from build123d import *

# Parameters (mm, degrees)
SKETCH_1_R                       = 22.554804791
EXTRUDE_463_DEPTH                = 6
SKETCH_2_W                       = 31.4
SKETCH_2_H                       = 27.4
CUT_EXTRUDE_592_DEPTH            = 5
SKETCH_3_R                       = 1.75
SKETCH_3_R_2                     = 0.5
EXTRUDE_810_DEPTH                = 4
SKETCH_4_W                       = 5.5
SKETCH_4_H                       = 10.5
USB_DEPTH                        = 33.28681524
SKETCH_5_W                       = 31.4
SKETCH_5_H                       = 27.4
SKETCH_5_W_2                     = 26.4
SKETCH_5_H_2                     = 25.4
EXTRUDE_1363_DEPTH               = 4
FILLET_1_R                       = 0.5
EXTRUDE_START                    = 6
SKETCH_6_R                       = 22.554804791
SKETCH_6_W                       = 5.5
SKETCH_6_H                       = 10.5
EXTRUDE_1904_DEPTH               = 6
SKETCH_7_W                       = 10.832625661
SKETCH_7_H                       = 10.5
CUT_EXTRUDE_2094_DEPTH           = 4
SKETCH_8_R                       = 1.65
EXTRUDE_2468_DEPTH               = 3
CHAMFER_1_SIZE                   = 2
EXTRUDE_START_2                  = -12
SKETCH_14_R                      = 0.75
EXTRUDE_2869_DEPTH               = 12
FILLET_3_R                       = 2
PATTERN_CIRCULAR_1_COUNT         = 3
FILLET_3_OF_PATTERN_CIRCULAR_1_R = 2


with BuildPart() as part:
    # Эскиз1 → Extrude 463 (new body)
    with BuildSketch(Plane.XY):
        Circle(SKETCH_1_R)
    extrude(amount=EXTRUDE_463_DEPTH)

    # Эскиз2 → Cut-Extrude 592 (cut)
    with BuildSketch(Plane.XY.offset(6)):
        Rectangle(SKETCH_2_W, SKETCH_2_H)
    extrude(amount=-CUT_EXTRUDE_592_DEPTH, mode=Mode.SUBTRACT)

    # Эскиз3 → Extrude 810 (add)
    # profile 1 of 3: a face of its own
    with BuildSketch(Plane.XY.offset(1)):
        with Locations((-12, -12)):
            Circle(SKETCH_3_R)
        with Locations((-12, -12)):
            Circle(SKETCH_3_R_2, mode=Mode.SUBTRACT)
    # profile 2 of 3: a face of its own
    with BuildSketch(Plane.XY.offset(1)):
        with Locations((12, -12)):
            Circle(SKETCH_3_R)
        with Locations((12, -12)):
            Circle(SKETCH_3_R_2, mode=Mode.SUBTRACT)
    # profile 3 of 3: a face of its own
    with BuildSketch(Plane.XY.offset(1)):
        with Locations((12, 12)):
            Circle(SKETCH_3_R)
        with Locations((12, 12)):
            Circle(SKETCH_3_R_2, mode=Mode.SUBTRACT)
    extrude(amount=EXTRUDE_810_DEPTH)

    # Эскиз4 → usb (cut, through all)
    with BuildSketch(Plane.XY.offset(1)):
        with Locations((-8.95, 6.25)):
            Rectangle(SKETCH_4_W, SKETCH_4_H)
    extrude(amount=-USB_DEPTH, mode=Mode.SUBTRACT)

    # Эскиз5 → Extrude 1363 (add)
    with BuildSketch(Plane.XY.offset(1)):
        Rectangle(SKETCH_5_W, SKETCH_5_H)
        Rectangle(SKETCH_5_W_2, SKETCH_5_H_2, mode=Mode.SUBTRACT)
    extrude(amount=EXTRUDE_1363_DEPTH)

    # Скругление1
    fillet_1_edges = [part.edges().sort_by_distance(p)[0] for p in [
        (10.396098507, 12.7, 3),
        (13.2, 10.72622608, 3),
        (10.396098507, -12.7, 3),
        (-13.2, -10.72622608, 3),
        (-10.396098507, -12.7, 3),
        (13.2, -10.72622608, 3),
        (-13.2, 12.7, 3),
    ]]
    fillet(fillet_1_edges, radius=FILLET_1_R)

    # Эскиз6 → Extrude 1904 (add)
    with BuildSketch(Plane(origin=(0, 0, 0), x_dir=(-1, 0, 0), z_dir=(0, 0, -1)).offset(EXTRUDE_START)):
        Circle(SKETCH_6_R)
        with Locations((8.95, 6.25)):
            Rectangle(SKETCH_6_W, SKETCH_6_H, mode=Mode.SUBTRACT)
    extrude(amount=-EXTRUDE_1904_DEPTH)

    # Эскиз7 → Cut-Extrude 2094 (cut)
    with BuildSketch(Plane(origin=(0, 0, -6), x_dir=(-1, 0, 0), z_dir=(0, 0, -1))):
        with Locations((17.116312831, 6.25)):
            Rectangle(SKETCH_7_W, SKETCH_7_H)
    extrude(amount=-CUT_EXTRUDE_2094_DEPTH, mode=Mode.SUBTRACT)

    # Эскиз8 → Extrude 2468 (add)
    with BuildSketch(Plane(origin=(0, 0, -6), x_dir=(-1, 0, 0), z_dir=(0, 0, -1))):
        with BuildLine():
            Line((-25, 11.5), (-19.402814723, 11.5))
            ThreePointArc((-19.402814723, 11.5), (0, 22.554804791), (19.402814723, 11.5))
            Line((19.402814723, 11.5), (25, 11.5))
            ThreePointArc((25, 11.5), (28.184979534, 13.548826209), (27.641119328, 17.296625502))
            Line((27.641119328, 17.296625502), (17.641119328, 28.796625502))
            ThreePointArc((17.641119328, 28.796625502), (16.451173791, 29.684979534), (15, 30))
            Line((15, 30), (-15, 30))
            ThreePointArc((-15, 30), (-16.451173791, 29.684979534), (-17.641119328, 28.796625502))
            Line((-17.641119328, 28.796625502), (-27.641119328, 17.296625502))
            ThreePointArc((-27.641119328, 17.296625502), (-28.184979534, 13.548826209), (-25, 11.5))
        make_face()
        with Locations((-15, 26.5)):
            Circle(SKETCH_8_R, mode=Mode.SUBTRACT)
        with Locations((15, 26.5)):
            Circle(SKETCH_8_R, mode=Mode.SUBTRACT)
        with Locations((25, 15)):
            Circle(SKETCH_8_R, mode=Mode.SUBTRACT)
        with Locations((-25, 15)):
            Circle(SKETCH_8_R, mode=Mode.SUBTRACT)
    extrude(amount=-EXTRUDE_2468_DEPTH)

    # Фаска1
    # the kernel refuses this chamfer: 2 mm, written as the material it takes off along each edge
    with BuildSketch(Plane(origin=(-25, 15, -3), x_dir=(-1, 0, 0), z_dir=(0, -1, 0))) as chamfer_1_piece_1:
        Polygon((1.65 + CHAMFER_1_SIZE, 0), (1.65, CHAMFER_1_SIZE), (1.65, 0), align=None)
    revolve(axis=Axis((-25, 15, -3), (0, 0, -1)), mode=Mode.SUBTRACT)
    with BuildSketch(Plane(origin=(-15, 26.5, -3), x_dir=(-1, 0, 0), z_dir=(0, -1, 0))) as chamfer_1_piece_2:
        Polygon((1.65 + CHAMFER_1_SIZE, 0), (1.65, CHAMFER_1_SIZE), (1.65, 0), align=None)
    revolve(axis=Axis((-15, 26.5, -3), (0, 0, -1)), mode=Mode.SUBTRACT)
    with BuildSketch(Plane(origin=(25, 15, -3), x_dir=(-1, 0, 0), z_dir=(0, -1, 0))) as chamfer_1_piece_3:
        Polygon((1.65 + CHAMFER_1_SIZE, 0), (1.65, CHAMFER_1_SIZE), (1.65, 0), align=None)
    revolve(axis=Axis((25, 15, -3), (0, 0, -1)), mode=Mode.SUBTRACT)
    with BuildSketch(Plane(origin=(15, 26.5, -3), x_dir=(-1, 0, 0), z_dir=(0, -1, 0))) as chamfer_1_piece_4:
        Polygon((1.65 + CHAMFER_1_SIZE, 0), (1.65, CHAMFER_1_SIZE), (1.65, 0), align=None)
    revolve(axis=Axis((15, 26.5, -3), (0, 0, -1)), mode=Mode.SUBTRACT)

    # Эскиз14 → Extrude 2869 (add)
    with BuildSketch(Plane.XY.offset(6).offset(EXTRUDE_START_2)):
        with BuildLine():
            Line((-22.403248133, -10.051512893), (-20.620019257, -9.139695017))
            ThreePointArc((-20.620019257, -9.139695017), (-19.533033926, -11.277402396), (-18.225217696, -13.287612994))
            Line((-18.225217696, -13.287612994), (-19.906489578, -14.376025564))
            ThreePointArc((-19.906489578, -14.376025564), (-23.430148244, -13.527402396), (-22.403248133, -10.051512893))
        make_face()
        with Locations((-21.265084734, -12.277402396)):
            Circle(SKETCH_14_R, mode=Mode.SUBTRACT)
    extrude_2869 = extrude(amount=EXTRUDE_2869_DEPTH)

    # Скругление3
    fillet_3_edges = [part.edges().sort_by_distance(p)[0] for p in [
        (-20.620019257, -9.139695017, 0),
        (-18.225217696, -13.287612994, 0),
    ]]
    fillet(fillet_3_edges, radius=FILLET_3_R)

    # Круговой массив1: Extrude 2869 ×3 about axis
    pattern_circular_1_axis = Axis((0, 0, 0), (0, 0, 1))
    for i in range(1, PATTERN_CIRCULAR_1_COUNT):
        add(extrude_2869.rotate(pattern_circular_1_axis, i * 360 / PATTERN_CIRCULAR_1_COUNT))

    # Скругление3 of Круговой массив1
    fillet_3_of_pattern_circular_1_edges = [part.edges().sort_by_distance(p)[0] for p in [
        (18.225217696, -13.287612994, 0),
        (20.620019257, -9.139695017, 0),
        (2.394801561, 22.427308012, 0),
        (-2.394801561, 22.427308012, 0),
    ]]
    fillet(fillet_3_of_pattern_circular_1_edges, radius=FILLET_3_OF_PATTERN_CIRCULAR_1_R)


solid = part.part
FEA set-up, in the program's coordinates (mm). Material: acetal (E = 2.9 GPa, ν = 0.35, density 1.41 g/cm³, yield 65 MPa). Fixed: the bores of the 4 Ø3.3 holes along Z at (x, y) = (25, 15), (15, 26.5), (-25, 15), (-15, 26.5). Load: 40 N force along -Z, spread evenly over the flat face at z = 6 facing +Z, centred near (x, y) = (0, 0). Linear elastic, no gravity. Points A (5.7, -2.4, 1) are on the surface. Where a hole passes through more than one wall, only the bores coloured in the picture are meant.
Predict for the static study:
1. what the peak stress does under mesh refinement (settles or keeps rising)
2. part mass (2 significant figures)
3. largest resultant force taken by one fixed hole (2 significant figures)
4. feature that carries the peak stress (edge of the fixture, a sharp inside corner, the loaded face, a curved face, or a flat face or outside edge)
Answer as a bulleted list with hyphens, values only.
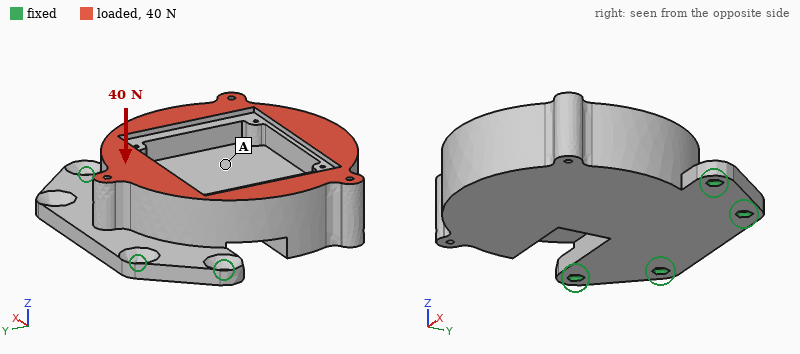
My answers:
- keeps rising
- 24 g
- 64 N
- edge of the fixture
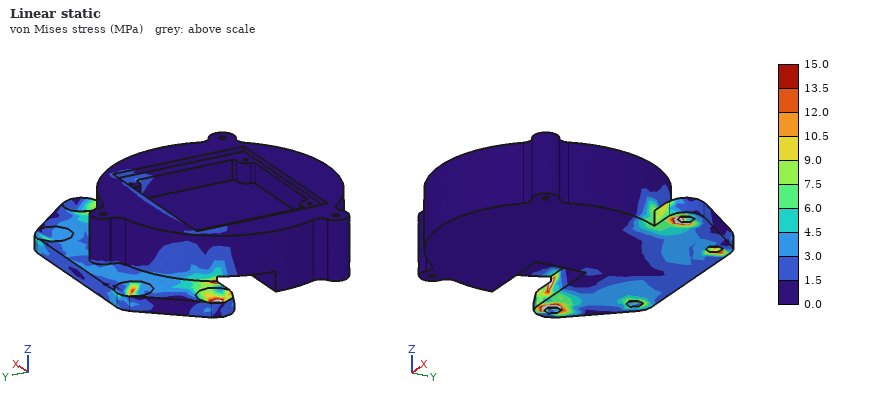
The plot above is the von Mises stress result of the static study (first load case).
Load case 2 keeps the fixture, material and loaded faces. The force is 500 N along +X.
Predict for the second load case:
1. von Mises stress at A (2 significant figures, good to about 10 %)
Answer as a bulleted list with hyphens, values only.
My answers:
- 5.5 MPa
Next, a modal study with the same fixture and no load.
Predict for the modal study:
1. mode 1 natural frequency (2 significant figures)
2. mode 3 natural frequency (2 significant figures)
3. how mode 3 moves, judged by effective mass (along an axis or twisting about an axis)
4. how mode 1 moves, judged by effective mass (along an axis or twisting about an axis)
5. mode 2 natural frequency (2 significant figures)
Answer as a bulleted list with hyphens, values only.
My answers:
- 380 Hz
- 1900 Hz
- along X
- along Z
- 1600 Hz
